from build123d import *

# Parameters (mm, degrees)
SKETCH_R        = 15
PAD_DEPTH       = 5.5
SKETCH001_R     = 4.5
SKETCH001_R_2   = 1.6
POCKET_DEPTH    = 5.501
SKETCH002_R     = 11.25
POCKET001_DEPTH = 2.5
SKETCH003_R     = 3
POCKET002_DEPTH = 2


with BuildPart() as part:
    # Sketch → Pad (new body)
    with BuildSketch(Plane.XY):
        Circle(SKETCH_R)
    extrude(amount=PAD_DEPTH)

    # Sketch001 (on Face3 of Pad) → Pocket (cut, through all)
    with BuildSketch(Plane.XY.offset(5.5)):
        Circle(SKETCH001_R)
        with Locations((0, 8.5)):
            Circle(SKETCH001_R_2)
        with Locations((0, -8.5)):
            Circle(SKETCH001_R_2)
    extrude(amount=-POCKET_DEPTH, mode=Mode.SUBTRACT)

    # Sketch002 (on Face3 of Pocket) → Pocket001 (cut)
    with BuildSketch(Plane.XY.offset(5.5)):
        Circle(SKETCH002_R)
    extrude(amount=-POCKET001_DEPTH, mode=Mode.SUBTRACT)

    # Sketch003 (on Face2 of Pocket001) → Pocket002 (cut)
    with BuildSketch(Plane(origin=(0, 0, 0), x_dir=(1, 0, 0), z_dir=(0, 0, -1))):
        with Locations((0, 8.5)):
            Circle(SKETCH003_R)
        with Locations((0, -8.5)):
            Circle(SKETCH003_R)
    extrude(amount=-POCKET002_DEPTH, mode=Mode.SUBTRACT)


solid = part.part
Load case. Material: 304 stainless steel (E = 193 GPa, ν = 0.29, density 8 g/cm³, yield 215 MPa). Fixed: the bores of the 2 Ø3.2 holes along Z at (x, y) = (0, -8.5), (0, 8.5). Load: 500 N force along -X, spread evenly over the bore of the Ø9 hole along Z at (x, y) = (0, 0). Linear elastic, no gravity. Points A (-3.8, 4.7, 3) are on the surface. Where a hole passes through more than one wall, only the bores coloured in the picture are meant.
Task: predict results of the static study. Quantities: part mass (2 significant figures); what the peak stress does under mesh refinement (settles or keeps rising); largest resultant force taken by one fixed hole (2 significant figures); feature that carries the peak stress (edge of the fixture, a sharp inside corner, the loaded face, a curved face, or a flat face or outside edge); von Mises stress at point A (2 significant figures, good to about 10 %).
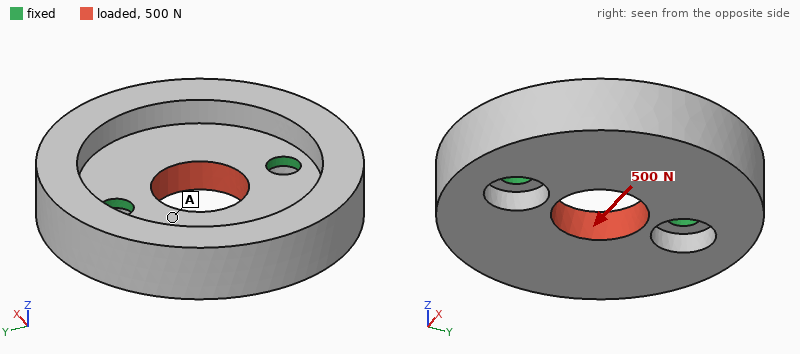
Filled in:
21 g
keeps rising
250 N
edge of the fixture
13 MPa
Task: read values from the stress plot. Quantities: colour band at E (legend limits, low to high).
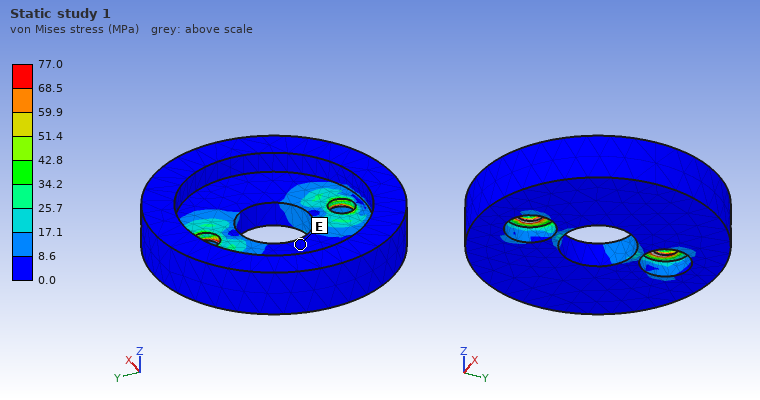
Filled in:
0.0 to 8.6 MPa
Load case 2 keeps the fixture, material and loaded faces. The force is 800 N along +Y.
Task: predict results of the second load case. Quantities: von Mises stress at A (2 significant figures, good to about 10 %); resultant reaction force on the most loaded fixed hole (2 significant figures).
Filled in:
20 MPa
400 N
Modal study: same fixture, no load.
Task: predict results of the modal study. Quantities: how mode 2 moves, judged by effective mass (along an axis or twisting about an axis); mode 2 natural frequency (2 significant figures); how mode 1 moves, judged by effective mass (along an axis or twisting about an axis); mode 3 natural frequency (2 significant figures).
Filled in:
along Z
12 kHz
twisting about Y
18 kHz
